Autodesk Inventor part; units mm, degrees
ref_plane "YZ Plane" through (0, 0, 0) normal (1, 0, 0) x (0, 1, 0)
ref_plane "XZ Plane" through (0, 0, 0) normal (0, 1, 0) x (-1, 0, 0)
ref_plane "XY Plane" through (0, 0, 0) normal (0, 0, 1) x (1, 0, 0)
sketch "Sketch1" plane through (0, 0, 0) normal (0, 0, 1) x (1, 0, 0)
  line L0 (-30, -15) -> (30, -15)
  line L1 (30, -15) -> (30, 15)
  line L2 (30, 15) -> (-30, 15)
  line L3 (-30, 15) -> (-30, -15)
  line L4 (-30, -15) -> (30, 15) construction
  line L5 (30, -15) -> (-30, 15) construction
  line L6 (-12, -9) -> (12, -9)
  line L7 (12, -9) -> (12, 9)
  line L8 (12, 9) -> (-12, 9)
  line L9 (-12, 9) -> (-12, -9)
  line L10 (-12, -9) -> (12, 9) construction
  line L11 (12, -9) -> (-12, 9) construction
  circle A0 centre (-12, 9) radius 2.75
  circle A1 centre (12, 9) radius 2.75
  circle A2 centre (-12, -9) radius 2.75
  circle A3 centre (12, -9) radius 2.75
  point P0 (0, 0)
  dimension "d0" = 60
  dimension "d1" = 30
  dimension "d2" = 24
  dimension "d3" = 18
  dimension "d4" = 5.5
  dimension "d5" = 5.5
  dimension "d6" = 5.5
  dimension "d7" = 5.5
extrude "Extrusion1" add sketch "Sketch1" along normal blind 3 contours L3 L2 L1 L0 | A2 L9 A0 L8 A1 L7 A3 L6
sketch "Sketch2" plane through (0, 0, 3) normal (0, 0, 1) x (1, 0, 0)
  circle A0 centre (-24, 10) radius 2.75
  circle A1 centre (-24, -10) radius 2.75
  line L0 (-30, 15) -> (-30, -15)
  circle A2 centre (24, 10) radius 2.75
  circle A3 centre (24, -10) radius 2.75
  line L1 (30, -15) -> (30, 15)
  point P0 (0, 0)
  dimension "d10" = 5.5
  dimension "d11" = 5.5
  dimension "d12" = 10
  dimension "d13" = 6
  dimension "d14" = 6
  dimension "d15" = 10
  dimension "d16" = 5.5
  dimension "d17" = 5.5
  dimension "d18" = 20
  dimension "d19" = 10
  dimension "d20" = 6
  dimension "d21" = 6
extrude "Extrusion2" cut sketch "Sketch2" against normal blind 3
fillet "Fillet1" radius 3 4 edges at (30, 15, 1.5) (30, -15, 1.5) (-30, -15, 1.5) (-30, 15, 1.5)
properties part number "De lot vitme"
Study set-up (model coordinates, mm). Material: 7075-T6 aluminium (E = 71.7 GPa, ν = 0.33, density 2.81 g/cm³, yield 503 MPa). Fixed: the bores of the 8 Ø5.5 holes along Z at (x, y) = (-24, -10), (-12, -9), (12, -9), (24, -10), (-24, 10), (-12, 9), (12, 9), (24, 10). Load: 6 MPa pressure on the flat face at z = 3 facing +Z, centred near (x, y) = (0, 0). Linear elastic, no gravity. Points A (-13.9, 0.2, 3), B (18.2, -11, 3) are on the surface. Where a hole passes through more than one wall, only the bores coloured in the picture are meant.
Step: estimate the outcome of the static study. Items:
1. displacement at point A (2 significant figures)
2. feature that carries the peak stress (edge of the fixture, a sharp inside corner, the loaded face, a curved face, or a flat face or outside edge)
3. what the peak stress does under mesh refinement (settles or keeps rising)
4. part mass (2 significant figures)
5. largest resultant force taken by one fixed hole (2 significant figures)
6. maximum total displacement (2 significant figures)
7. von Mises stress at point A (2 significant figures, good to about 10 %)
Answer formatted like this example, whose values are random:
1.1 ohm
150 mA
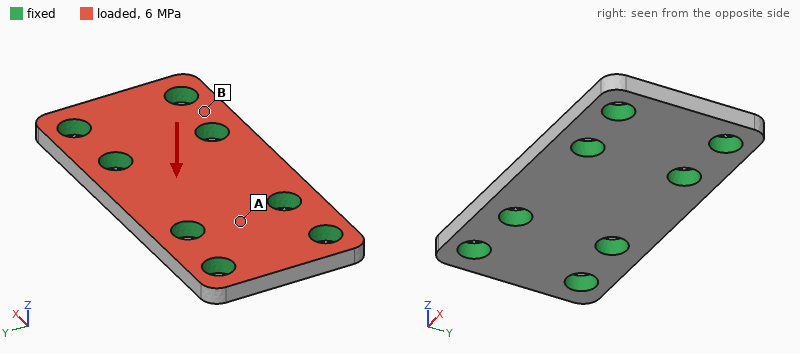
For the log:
6.8 µm
edge of the fixture
keeps rising
14 g
1.5 kN
27 µm
42 MPa
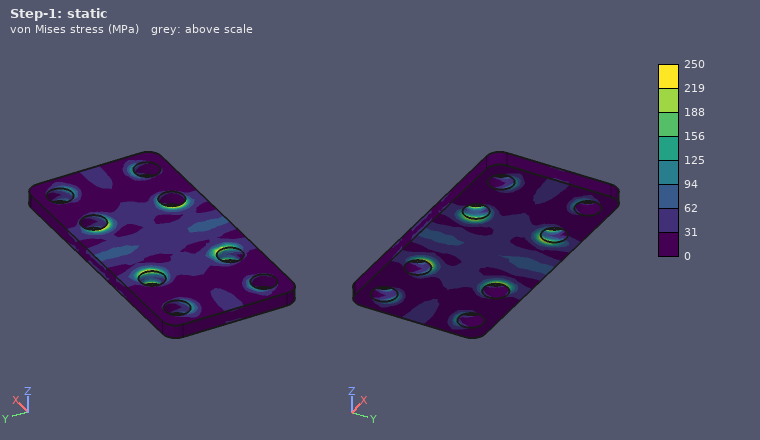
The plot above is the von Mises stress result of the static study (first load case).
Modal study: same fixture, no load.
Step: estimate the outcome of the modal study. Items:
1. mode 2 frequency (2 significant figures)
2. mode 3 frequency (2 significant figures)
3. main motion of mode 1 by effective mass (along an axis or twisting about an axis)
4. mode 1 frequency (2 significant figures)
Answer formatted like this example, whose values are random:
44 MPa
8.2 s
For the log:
35 kHz
39 kHz
along Z
30 kHz
